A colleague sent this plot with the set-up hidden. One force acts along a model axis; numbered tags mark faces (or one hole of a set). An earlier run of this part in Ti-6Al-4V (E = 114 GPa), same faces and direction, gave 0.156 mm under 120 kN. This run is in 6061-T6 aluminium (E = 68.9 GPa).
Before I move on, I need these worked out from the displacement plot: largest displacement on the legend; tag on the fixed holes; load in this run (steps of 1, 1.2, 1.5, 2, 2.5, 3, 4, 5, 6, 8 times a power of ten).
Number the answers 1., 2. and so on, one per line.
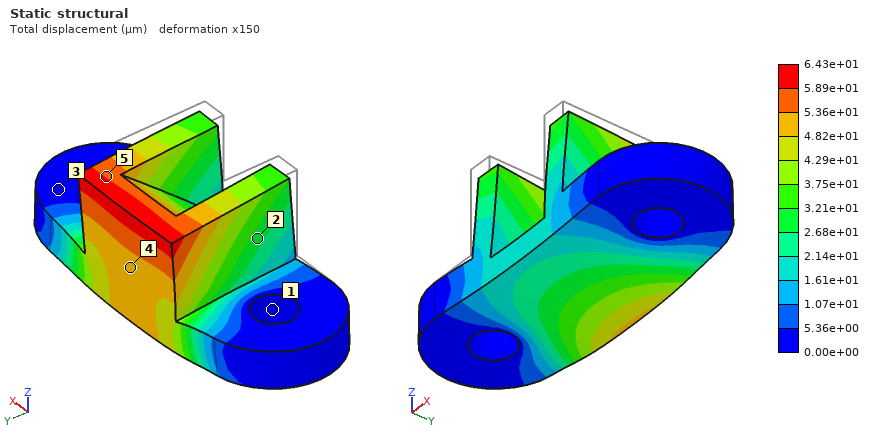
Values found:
1. 6.43e+01 µm
2. 1
3. 30 kN
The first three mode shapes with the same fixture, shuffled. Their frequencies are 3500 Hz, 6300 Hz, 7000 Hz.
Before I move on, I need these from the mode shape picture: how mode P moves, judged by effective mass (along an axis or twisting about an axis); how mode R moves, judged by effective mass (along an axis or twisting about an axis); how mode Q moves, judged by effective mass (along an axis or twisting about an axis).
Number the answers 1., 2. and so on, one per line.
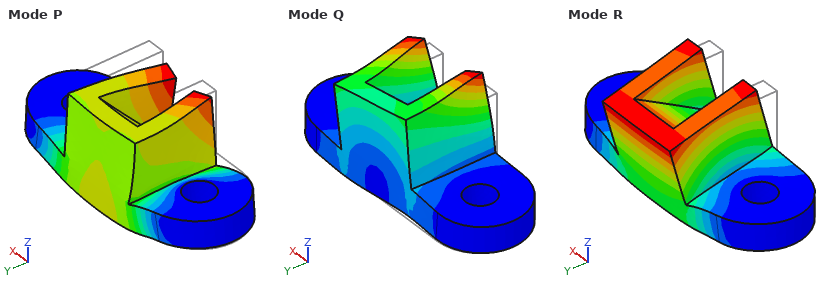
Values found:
1. along Z
2. along Y
3. along X
